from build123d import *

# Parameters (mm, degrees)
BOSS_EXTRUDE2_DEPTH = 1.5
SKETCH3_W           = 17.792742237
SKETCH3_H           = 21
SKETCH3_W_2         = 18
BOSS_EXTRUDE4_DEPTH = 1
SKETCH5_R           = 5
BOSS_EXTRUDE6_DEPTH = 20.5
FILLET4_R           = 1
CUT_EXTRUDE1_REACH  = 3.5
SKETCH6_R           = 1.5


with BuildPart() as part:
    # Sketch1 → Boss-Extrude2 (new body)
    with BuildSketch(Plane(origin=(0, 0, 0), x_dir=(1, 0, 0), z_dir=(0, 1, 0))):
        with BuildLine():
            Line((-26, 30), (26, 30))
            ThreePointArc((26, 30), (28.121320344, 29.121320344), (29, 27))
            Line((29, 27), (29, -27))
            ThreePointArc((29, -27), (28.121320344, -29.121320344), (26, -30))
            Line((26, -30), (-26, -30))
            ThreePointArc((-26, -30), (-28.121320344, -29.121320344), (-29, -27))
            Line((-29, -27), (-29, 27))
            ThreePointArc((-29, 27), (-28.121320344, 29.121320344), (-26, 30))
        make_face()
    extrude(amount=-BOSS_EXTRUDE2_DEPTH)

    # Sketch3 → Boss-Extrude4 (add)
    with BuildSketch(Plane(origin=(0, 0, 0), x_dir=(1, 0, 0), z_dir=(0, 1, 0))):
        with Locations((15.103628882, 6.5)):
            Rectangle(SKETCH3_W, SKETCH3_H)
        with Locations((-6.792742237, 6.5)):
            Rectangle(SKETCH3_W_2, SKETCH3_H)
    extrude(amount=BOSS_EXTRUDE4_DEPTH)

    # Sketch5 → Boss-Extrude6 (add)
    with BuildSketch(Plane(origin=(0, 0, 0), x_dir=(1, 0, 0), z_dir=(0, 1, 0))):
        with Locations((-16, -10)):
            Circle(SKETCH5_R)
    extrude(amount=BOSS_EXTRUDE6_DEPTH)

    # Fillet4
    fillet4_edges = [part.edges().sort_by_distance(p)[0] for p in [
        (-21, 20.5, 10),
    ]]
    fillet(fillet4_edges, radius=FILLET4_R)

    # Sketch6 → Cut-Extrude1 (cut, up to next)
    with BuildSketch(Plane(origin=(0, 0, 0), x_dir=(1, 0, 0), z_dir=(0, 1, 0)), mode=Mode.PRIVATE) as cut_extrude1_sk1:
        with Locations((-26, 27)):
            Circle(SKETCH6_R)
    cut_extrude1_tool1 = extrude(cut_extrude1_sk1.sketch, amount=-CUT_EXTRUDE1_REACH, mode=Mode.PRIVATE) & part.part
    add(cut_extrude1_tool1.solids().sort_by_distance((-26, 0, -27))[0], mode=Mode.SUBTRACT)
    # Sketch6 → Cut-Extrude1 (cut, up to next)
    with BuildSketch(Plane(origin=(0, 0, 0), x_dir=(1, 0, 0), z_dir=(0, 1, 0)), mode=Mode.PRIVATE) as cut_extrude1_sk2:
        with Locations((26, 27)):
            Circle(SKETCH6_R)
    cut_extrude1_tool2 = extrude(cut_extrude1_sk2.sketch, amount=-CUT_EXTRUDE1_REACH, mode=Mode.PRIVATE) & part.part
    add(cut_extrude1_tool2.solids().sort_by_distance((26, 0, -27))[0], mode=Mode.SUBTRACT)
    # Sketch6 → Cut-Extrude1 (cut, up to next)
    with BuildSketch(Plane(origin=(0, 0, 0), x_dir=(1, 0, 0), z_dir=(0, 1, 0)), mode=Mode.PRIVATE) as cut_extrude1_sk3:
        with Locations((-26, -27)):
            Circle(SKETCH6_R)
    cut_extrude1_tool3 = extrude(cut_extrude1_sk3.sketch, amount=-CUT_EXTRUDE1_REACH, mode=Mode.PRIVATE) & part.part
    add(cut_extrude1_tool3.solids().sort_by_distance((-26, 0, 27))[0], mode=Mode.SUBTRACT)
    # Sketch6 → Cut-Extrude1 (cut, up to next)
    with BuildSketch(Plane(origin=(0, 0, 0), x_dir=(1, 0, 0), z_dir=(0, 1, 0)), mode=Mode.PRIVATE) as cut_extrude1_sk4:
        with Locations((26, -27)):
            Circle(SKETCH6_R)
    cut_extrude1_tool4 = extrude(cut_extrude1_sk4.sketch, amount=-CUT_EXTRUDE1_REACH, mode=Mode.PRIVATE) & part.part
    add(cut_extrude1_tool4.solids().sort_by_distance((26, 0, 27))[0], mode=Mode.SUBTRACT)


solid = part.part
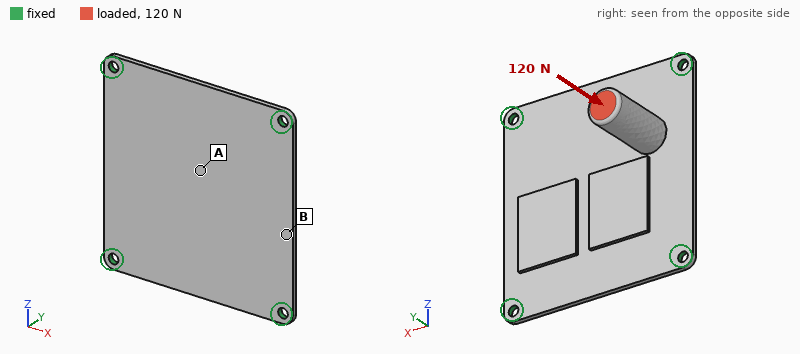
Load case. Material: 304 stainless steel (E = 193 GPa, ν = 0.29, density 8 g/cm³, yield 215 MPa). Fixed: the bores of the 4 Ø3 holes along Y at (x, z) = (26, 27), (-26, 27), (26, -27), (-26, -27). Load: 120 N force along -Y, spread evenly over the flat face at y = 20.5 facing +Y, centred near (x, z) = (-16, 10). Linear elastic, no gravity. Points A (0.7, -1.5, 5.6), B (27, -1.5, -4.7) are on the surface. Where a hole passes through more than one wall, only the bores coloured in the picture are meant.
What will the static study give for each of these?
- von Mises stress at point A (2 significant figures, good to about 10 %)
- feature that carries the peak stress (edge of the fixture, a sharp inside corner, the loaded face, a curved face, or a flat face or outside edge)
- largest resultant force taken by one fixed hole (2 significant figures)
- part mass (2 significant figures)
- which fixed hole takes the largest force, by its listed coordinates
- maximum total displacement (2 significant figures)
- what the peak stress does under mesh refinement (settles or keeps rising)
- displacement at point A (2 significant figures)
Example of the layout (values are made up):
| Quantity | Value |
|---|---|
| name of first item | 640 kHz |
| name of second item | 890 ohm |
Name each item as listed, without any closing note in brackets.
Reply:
| Quantity | Value |
|---|---|
| von Mises stress at point A | 21 MPa |
| feature that carries the peak stress | edge of the fixture |
| largest resultant force taken by one fixed hole | 74 N |
| part mass | 60 g |
| which fixed hole takes the largest force, by its listed coordinates | (-26, 27) |
| maximum total displacement | 48 µm |
| what the peak stress does under mesh refinement | keeps rising |
| displacement at point A | 34 µm |
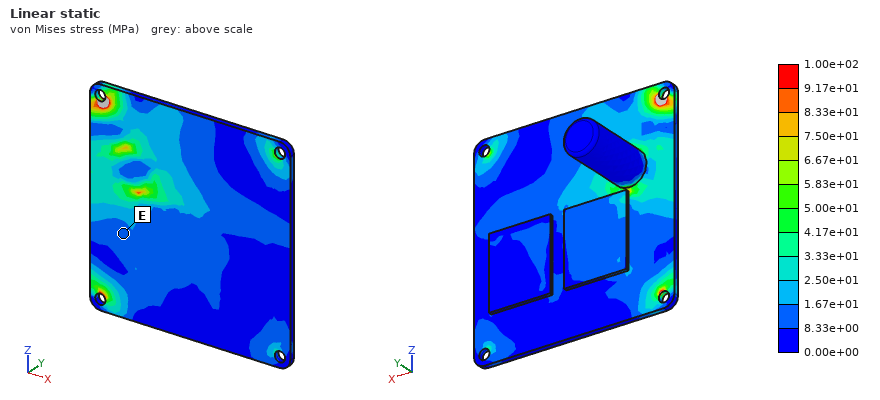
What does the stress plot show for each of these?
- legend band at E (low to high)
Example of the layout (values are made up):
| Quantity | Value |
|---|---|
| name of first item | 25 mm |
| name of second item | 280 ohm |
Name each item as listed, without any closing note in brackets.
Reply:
| Quantity | Value |
|---|---|
| legend band at E | 8.33e+00 to 1.67e+01 MPa |
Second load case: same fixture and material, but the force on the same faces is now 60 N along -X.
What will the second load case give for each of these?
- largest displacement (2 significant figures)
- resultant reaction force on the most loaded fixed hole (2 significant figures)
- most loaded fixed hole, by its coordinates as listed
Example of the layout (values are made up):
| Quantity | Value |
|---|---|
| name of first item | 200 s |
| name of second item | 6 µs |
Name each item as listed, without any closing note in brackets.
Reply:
| Quantity | Value |
|---|---|
| largest displacement | 58 µm |
| resultant reaction force on the most loaded fixed hole | 32 N |
| most loaded fixed hole, by its coordinates as listed | (26, -27) |
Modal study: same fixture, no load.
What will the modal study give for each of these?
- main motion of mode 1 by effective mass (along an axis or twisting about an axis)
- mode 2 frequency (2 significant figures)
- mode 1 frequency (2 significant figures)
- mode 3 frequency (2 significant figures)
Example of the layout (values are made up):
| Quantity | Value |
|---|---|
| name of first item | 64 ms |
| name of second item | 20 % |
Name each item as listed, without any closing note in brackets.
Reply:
| Quantity | Value |
|---|---|
| main motion of mode 1 by effective mass | along Y |
| mode 2 frequency | 2100 Hz |
| mode 1 frequency | 1500 Hz |
| mode 3 frequency | 2900 Hz |
